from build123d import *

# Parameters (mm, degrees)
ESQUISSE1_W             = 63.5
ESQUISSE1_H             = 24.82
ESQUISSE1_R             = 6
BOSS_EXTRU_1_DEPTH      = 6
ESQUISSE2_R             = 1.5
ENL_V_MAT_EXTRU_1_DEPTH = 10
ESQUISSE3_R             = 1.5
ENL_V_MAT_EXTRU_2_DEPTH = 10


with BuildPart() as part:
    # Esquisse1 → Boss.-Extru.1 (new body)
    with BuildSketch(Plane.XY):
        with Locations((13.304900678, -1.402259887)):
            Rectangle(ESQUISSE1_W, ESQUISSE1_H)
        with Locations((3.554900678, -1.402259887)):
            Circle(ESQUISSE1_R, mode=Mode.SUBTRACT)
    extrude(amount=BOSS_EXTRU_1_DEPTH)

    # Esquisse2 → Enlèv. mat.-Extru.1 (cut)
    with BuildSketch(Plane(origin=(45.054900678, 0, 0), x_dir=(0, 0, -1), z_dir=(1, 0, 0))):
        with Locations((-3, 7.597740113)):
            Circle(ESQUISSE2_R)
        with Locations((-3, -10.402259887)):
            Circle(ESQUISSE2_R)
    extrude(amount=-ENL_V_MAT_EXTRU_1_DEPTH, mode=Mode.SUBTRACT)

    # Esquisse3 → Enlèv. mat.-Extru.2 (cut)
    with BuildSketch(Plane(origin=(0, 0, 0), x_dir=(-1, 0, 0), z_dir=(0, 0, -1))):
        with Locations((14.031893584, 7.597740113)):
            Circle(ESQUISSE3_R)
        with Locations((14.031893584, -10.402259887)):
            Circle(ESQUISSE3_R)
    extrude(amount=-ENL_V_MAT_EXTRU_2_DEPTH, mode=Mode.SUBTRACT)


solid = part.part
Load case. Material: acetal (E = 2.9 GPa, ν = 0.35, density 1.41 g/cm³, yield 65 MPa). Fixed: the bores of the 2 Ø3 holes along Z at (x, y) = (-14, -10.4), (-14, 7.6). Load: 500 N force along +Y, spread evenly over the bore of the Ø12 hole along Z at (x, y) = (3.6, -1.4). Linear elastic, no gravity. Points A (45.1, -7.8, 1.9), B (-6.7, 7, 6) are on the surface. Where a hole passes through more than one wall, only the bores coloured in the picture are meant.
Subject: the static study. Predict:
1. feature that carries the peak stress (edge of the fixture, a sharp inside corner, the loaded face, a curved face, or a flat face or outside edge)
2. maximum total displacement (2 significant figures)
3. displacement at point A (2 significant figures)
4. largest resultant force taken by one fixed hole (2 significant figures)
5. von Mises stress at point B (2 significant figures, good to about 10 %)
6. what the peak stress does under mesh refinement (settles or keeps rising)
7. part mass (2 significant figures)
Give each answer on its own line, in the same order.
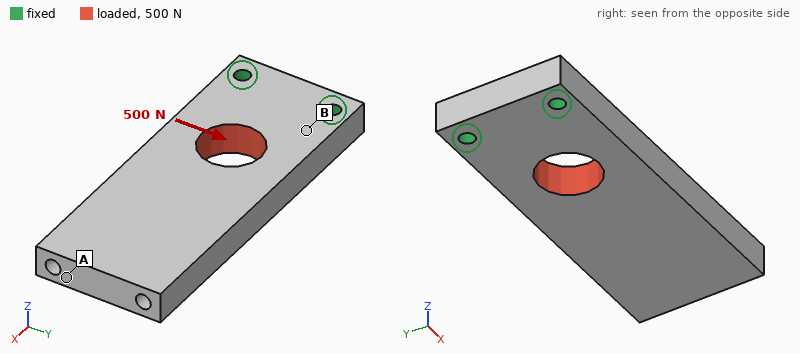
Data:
edge of the fixture
0.34 mm
0.34 mm
510 N
6.1 MPa
keeps rising
12 g
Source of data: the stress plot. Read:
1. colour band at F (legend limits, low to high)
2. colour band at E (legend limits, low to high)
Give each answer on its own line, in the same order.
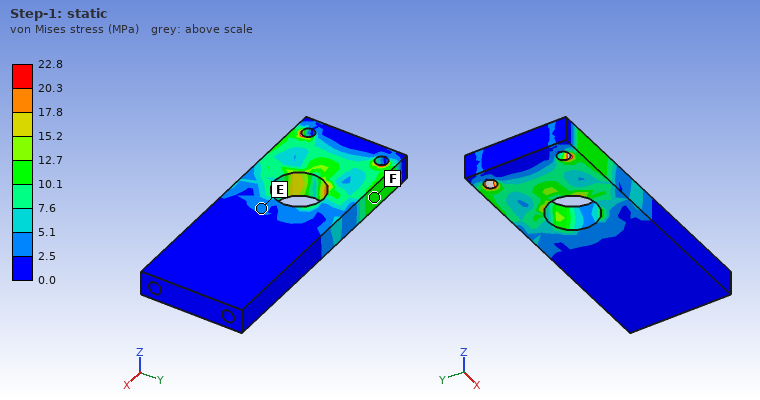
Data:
10.1 to 12.7 MPa
2.5 to 5.1 MPa
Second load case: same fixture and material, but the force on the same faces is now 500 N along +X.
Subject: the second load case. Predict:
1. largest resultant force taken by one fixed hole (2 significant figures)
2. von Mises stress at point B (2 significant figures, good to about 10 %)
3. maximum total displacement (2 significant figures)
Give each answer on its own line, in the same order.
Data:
250 N
4.5 MPa
40 µm
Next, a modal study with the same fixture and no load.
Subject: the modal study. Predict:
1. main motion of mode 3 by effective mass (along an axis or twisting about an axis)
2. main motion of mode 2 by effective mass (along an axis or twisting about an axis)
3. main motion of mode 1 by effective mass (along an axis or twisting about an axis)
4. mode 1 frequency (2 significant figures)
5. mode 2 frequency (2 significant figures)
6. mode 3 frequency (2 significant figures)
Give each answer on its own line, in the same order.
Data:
twisting about X
along Y
along Z
350 Hz
1400 Hz
1600 Hz
